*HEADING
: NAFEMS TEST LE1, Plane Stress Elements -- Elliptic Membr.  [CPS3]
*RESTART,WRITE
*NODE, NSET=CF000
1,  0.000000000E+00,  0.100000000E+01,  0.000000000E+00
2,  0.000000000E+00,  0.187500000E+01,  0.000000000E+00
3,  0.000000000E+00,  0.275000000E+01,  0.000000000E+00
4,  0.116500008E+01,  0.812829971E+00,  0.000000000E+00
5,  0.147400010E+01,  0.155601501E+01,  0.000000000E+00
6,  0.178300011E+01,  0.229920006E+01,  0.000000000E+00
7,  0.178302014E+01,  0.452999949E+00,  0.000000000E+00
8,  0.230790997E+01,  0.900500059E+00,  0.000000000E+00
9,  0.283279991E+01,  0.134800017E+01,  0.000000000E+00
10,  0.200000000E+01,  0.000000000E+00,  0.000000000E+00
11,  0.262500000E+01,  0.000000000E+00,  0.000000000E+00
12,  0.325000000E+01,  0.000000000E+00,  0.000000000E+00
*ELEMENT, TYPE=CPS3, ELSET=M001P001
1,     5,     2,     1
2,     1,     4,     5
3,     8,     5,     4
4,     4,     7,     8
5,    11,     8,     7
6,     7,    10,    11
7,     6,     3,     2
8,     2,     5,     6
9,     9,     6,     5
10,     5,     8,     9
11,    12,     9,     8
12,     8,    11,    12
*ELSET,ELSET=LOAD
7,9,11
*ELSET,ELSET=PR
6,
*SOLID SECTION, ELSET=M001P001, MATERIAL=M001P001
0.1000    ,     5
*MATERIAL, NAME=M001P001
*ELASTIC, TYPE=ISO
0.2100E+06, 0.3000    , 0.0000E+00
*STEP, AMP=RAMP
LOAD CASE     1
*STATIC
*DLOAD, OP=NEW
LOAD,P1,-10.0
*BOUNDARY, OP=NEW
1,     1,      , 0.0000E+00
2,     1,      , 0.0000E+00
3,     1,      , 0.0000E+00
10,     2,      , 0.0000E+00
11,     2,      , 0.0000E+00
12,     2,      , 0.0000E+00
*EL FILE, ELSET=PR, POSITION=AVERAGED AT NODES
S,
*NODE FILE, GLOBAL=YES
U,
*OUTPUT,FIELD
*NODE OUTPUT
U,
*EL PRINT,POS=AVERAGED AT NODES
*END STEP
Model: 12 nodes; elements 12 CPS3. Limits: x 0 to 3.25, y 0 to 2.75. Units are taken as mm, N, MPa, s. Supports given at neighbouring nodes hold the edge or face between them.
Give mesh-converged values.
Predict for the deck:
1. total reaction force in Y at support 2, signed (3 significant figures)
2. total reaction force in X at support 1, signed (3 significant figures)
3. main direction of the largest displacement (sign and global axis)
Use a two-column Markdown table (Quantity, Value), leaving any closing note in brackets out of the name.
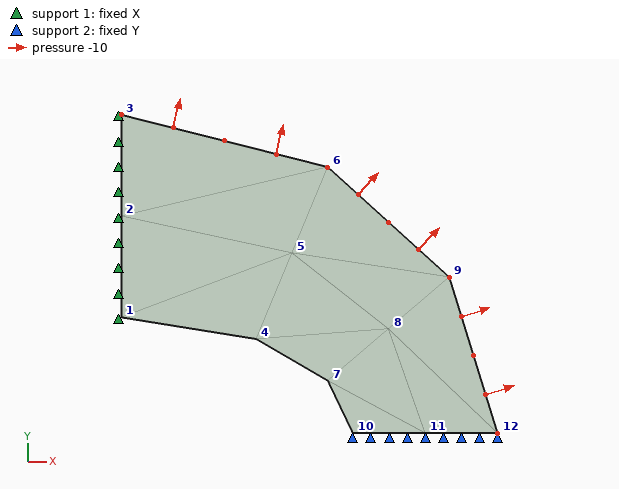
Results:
| Quantity | Value |
|---|---|
| total reaction force in Y at support 2, signed | -3.25 N |
| total reaction force in X at support 1, signed | -2.75 N |
| main direction of the largest displacement | +Y |
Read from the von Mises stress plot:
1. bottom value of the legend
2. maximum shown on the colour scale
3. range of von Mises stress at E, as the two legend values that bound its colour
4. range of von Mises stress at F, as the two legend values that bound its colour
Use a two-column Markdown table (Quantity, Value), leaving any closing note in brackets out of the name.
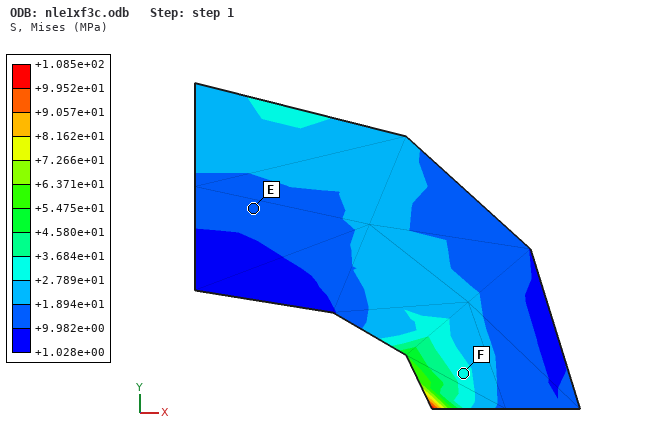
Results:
| Quantity | Value |
|---|---|
| bottom value of the legend | +1.028e+00 MPa |
| maximum shown on the colour scale | +1.085e+02 MPa |
| range of von Mises stress at E, as the two legend values that bound its colour | +9.982e+00 to +1.894e+01 MPa |
| range of von Mises stress at F, as the two legend values that bound its colour | +2.789e+01 to +3.684e+01 MPa |
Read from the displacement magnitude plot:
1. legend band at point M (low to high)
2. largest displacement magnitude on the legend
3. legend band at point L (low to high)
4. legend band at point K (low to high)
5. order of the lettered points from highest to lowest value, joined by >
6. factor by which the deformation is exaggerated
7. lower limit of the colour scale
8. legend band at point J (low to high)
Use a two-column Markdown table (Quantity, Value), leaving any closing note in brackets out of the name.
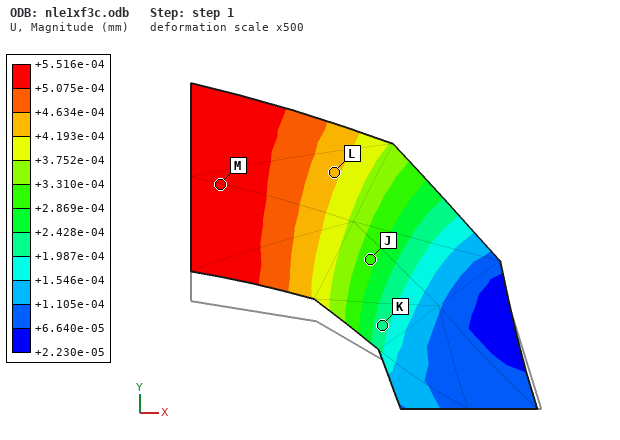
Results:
| Quantity | Value |
|---|---|
| legend band at point M | +5.075e-04 to +5.516e-04 mm |
| largest displacement magnitude on the legend | +5.516e-04 mm |
| legend band at point L | +4.193e-04 to +4.634e-04 mm |
| legend band at point K | +1.987e-04 to +2.428e-04 mm |
| order of the lettered points from highest to lowest value, joined by > | M > L > J > K |
| factor by which the deformation is exaggerated | 500 |
| lower limit of the colour scale | +2.230e-05 mm |
| legend band at point J | +2.869e-04 to +3.310e-04 mm |
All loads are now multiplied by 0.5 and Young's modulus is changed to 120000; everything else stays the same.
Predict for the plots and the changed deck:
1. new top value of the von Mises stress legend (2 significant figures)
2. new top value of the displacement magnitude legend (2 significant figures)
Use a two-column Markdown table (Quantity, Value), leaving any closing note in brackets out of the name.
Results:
| Quantity | Value |
|---|---|
| new top value of the von Mises stress legend | 54 MPa |
| new top value of the displacement magnitude legend | 4.8e-04 mm |
